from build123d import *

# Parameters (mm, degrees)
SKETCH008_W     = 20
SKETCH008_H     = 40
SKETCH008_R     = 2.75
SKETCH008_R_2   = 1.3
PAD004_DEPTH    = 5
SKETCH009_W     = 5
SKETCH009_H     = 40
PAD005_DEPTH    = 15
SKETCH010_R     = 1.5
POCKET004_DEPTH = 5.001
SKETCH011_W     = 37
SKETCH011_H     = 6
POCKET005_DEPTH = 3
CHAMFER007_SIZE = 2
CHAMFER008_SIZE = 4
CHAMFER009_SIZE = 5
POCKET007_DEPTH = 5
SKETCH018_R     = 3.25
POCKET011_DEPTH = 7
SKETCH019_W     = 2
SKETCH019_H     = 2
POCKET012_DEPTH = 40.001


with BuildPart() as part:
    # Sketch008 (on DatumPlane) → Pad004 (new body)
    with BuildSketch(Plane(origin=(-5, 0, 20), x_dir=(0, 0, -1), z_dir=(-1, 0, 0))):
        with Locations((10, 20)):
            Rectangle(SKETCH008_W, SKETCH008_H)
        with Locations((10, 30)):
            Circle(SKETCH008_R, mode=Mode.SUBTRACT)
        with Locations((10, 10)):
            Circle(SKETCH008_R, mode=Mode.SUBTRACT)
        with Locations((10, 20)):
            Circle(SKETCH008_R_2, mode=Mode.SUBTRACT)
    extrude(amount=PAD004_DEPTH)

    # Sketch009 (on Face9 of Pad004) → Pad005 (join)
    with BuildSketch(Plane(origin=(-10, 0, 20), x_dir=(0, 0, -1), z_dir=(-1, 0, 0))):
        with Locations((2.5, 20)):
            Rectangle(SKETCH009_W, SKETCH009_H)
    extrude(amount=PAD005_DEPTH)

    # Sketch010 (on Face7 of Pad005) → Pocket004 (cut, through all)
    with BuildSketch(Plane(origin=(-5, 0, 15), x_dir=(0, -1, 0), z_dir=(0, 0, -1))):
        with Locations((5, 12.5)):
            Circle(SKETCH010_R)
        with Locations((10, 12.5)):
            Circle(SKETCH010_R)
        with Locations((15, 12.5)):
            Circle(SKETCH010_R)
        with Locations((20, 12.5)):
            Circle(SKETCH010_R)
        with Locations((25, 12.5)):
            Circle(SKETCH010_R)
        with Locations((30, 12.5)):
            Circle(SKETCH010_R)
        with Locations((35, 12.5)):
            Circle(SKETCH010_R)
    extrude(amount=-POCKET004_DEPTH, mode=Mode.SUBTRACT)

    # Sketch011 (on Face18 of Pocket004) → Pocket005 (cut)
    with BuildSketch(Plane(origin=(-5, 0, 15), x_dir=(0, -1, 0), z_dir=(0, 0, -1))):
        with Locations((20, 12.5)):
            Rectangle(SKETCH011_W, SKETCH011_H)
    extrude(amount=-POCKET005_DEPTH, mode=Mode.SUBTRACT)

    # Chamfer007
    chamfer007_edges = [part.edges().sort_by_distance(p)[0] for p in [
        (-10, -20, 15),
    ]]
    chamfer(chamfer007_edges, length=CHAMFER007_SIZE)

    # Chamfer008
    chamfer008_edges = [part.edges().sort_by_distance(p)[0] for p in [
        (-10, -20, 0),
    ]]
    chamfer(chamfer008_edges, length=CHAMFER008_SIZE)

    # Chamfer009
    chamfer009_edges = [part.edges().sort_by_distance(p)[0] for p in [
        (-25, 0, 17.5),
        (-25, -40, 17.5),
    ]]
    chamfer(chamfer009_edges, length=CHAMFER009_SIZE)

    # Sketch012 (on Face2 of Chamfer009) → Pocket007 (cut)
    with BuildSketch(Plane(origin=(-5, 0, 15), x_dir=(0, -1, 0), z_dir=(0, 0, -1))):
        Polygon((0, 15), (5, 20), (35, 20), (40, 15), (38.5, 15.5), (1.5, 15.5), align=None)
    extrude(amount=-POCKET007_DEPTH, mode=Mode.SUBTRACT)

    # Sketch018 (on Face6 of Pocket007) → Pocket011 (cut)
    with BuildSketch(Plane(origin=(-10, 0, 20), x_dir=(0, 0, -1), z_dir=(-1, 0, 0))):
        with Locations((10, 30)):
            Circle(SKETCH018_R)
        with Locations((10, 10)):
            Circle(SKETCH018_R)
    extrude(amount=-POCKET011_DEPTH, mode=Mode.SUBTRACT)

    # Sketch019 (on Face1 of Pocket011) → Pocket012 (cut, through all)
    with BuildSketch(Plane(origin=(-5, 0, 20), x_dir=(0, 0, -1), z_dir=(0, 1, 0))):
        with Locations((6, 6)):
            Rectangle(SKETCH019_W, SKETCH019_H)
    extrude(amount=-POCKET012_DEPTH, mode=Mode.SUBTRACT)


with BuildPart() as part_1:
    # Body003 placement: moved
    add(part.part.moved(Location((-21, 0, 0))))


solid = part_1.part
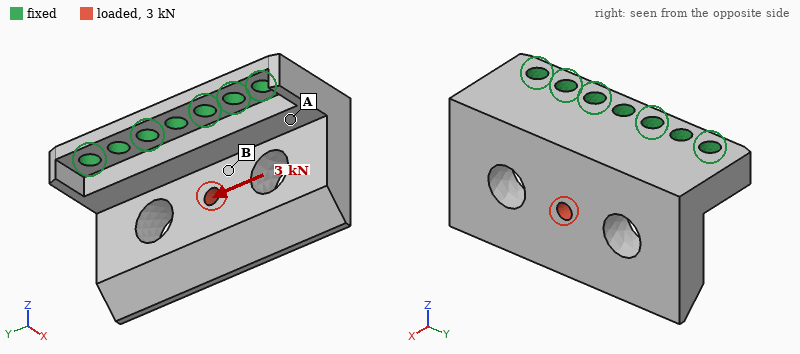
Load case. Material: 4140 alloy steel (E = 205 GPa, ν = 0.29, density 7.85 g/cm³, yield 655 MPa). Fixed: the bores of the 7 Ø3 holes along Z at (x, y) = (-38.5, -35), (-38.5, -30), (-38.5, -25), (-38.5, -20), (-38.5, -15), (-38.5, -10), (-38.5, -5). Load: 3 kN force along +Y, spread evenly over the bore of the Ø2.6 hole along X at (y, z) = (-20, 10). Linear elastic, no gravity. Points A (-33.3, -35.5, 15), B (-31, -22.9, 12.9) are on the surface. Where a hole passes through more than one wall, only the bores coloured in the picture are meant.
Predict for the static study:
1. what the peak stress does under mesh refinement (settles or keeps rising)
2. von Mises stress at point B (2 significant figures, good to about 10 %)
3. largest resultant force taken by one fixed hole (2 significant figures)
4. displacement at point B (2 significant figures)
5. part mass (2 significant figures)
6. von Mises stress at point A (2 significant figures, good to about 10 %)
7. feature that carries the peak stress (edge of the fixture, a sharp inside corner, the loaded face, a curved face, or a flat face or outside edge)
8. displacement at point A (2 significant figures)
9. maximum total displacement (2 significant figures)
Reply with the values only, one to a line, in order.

keeps rising
99 MPa
990 N
9.1 µm
37 g
51 MPa
edge of the fixture
9.2 µm
31 µm
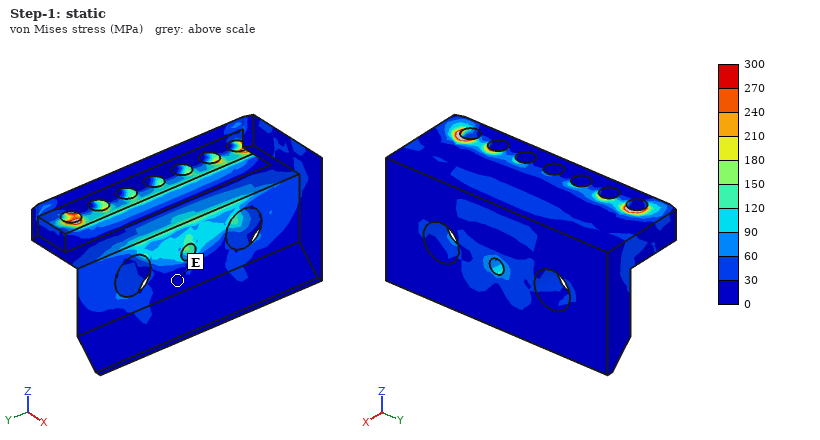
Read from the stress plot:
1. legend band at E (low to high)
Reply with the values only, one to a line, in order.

0 to 30 MPa
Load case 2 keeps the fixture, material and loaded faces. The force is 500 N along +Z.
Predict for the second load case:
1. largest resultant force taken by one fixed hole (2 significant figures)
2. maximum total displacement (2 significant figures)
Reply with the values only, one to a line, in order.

84 N
37 µm
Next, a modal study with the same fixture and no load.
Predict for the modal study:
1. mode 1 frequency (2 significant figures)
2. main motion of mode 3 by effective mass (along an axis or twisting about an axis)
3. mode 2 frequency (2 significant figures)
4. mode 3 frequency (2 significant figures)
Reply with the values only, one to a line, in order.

3600 Hz
along Y
8600 Hz
17 kHz
